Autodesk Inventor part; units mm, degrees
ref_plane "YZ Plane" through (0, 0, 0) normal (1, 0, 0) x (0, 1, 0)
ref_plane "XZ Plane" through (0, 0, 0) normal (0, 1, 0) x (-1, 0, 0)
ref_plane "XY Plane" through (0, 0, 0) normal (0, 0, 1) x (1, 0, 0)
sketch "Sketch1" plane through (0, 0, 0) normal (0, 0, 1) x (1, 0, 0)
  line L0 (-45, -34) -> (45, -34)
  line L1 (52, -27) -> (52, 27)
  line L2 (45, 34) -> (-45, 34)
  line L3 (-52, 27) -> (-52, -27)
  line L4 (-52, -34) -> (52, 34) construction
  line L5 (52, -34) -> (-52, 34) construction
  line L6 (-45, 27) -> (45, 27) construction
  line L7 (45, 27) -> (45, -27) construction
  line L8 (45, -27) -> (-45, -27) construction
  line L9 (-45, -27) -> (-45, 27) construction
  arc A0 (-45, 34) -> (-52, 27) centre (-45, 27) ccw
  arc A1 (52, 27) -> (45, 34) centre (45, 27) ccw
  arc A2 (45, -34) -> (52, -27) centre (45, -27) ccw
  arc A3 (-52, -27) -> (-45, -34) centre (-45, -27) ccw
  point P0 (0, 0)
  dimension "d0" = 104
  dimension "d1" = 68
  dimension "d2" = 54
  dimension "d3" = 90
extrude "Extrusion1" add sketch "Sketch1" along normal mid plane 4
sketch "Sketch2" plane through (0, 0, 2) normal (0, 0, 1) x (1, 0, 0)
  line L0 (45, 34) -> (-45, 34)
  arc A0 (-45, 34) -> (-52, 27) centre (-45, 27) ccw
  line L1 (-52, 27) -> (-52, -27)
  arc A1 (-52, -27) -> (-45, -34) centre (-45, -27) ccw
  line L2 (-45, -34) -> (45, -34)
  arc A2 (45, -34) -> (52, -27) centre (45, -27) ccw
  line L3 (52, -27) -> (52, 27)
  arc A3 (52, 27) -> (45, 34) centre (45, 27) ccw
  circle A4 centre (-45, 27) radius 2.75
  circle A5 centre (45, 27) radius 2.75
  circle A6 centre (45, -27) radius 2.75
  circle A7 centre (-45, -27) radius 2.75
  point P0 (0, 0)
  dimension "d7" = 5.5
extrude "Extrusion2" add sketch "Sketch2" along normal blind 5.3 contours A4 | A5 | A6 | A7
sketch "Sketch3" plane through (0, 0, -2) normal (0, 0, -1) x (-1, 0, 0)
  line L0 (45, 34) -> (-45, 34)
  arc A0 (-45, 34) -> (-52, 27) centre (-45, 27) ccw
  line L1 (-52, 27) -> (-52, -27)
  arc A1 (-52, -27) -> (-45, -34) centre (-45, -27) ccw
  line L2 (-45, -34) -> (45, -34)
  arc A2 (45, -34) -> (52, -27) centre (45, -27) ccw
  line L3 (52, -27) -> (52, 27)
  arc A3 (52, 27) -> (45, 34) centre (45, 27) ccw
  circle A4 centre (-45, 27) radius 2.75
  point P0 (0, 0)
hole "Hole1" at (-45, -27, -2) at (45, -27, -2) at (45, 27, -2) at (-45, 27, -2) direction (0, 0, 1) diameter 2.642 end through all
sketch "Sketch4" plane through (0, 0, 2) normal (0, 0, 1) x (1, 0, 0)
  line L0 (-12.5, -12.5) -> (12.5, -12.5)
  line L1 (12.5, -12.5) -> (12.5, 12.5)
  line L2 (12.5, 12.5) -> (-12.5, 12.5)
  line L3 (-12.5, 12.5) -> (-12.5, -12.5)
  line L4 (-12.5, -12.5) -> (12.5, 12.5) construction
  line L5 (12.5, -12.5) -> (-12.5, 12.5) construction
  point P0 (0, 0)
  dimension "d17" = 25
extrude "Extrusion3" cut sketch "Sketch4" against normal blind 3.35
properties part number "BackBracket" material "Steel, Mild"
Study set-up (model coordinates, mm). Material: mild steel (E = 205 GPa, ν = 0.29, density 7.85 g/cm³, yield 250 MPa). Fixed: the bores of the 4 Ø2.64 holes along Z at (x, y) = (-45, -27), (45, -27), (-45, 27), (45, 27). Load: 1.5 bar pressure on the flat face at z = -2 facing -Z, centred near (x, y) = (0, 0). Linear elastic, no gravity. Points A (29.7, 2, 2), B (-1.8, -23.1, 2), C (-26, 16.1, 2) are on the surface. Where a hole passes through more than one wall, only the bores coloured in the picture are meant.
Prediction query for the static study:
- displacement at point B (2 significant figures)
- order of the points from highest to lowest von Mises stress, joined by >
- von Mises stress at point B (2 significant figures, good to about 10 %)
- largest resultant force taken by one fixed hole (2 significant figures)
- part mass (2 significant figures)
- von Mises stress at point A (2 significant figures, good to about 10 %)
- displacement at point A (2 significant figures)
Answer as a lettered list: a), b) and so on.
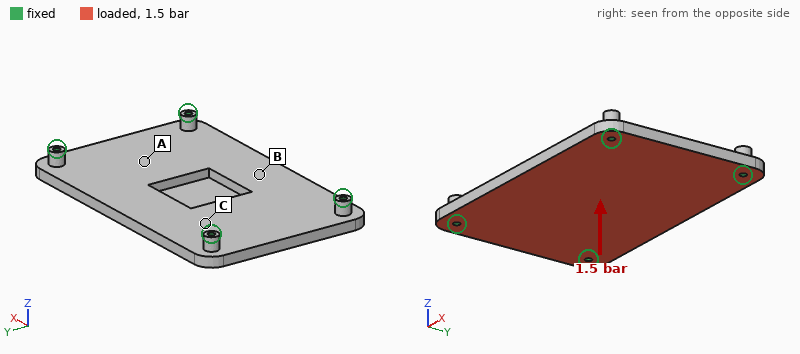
a) 37 µm
b) B > A > C
c) 27 MPa
d) 290 N
e) 210 g
f) 12 MPa
g) 20 µm
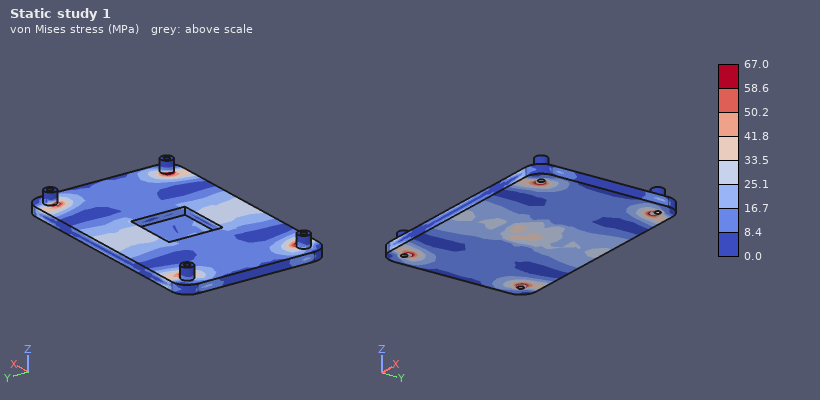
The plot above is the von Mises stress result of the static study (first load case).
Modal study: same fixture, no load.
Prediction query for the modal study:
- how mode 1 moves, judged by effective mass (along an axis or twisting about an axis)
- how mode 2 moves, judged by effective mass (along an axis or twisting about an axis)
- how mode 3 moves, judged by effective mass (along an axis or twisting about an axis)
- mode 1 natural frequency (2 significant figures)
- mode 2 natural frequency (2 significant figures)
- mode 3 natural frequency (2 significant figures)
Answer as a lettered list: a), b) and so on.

a) along Z
b) twisting about X
c) twisting about Y
d) 2200 Hz
e) 3300 Hz
f) 5200 Hz
